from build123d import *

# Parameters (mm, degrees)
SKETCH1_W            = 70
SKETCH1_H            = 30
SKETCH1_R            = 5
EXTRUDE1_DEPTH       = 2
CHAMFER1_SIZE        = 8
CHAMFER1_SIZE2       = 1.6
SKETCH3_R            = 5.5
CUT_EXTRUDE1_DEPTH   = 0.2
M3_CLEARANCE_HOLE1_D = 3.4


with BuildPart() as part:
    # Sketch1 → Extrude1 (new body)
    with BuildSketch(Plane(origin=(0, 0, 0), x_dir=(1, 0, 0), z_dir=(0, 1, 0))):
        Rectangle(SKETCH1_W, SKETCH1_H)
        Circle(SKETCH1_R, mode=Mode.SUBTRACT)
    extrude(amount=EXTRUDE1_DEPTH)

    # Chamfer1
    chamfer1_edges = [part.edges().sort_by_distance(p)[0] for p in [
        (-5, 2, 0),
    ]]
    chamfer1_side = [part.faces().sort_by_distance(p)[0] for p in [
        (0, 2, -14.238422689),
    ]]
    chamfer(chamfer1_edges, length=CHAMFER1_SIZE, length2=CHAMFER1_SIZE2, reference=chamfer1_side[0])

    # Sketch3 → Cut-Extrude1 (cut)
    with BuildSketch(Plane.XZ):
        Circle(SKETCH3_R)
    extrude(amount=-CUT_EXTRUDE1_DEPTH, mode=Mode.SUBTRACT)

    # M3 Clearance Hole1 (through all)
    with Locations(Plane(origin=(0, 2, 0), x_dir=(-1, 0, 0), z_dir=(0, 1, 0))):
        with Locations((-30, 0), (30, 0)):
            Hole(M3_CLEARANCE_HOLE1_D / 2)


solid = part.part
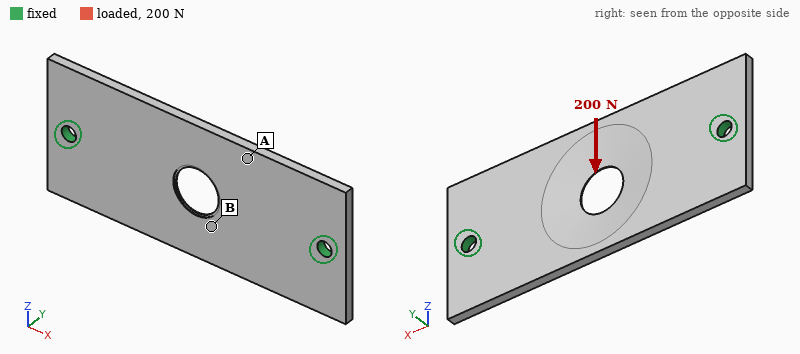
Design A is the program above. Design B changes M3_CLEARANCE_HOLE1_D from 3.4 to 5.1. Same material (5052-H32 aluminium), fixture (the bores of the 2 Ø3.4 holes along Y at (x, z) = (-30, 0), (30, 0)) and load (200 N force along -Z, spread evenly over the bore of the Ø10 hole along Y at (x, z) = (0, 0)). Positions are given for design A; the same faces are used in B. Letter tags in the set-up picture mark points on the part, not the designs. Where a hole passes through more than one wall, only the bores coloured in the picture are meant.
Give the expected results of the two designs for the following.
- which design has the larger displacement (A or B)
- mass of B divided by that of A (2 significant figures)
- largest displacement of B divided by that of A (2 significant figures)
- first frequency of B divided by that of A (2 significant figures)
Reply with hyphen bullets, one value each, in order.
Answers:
- A
- 0.99
- 0.87
- 1.1
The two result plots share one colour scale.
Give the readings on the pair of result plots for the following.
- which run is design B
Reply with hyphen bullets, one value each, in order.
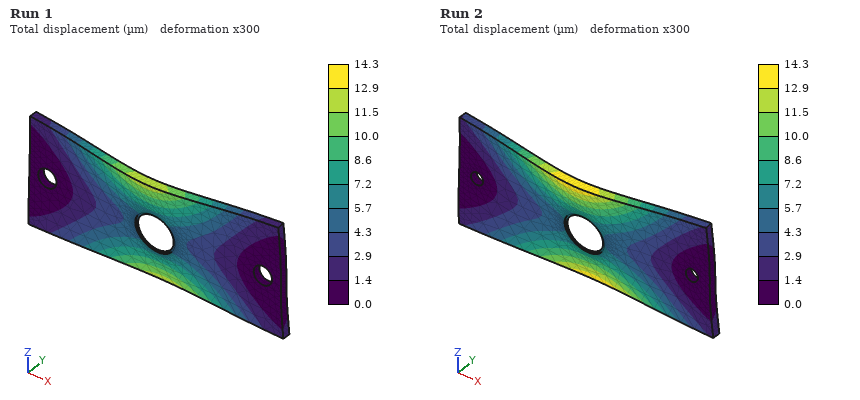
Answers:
- Run 1
